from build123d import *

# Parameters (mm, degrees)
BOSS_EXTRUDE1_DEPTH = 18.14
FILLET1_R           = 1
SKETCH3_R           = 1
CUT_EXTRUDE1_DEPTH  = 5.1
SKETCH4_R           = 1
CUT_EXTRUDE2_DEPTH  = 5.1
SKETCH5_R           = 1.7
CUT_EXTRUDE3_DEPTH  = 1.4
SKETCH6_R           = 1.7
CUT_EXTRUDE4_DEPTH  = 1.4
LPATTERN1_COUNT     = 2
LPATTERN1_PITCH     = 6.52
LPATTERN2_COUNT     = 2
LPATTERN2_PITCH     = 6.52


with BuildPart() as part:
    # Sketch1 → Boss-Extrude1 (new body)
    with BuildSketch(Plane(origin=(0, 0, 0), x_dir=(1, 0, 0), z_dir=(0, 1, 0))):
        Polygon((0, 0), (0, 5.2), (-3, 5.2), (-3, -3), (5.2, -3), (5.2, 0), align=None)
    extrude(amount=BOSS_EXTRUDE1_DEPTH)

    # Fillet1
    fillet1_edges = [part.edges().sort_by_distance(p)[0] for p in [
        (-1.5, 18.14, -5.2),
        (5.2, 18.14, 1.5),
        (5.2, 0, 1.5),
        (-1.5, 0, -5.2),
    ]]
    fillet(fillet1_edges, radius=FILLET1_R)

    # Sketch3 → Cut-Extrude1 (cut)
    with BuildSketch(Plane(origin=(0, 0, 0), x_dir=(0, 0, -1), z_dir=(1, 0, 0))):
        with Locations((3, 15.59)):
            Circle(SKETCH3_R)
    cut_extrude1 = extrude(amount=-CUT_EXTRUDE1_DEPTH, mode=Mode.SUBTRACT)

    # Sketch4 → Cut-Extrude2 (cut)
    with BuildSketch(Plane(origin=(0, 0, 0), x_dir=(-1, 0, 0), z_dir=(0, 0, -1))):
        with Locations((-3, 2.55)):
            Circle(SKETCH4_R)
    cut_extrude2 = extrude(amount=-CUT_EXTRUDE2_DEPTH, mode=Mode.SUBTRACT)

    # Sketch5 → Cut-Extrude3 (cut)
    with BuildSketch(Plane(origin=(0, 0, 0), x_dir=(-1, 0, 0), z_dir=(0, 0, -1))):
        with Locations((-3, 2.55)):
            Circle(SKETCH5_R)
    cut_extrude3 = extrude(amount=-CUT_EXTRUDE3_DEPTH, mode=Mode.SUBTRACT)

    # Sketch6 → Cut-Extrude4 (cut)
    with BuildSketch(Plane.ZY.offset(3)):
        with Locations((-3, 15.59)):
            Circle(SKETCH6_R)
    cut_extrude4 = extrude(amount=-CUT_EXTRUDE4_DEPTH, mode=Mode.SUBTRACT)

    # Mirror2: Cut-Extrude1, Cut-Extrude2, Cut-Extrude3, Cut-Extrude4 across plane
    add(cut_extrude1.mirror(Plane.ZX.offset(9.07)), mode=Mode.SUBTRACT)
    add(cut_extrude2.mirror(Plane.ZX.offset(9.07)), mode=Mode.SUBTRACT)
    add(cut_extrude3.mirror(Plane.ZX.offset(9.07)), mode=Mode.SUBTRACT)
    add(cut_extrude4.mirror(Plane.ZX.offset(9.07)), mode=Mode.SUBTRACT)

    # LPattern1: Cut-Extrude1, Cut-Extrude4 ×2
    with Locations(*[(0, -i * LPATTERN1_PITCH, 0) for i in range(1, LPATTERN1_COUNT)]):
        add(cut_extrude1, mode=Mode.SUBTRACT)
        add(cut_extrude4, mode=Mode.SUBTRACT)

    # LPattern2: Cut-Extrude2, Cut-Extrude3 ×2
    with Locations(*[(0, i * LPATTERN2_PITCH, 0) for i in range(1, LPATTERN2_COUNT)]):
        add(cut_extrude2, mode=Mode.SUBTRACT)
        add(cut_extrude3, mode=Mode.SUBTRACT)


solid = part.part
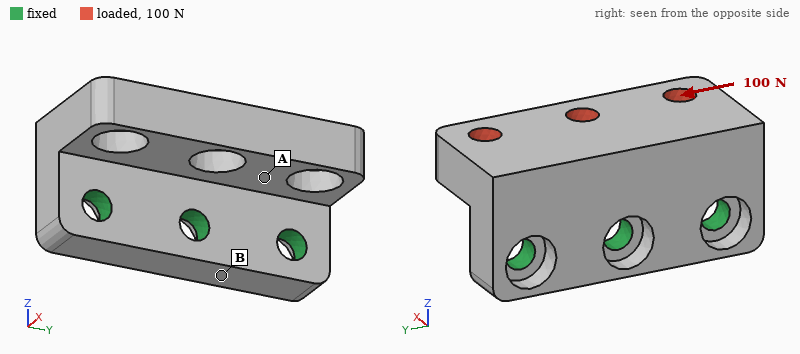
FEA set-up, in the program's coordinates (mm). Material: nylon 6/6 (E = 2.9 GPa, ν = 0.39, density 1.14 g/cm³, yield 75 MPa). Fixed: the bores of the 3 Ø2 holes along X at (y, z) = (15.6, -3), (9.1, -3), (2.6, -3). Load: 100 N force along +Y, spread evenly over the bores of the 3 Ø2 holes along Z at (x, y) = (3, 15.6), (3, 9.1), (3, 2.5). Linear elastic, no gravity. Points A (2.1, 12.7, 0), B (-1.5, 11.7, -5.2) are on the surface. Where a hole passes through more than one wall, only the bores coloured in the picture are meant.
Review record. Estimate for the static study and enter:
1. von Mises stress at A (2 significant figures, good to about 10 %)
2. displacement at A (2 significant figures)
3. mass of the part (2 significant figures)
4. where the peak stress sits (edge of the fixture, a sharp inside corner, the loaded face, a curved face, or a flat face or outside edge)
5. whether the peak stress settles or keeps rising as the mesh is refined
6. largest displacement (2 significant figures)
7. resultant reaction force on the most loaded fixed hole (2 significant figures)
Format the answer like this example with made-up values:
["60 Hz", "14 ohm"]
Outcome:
["5.8 MPa", "33 µm", "0.71 g", "edge of the fixture", "keeps rising", "69 µm", "52 N"]
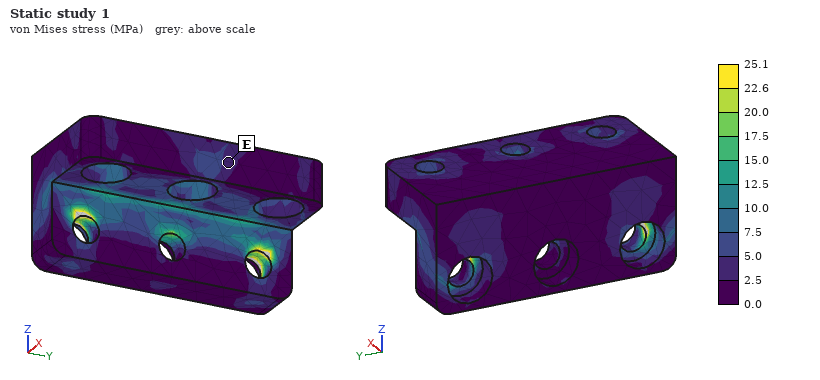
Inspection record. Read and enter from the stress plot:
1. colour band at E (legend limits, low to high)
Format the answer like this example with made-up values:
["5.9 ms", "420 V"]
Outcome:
["2.5 to 5.0 MPa"]
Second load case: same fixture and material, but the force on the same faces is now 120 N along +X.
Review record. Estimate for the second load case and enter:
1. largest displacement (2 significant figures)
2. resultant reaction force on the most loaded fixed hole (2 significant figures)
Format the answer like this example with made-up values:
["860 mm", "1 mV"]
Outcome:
["0.23 mm", "42 N"]
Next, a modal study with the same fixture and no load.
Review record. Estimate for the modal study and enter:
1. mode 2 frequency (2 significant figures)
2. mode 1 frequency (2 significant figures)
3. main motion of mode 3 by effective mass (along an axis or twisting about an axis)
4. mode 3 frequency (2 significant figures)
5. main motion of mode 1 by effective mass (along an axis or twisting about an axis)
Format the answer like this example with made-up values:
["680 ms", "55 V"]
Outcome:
["10 kHz", "6500 Hz", "along Y", "18 kHz", "along X"]
